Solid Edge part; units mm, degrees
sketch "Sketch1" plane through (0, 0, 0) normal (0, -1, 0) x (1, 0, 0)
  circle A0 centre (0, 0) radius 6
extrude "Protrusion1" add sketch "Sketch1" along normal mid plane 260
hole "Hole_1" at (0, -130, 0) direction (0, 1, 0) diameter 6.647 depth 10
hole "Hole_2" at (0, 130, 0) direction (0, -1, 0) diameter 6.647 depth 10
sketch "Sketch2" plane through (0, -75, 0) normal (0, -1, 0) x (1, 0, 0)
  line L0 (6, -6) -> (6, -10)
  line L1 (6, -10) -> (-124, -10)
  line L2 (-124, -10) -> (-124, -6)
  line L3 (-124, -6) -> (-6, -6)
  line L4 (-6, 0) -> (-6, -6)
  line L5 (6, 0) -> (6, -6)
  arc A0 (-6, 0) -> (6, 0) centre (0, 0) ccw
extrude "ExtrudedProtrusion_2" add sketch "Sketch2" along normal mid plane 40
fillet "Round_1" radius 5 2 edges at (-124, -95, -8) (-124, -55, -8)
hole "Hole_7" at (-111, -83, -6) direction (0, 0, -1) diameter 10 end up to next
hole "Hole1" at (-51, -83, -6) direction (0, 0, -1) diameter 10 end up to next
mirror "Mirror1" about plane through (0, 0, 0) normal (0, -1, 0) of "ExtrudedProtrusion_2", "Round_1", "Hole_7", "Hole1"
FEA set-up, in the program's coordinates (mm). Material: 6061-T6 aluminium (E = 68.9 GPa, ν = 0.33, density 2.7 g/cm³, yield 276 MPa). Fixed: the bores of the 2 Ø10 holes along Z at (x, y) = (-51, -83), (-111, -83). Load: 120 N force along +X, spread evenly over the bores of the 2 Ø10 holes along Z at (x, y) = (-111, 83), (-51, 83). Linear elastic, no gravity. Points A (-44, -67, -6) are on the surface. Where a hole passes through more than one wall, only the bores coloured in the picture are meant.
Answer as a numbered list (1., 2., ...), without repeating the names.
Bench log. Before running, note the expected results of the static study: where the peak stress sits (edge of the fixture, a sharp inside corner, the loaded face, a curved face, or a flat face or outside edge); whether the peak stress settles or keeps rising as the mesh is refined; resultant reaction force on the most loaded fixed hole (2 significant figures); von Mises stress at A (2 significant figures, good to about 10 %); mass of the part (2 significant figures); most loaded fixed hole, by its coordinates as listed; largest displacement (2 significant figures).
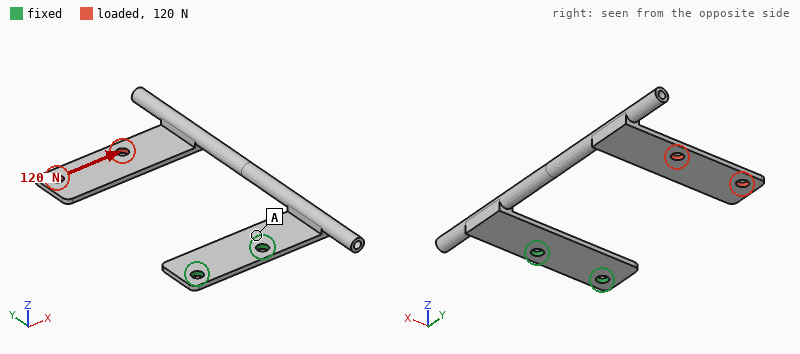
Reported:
1. a sharp inside corner
2. keeps rising
3. 360 N
4. 8.9 MPa
5. 190 g
6. (-111, -83)
7. 3.2 mm
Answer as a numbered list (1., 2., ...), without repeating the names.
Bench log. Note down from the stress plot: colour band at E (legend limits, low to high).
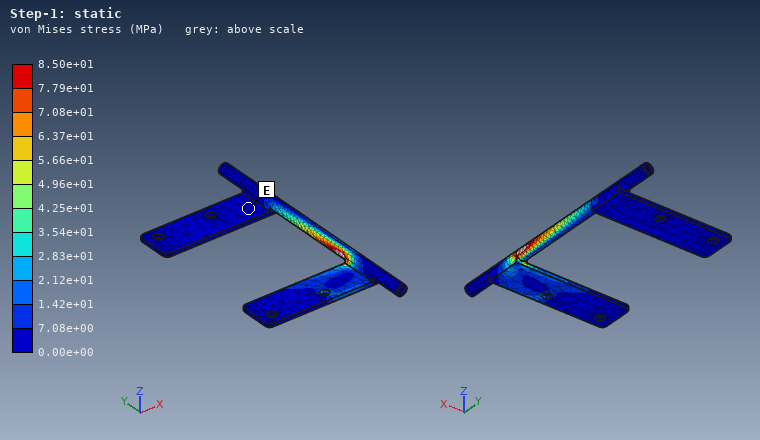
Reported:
1. 0.00e+00 to 7.08e+00 MPa
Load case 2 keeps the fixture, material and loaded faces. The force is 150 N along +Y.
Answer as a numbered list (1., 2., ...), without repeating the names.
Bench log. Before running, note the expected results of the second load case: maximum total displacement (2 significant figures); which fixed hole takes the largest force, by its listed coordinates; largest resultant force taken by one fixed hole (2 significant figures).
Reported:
1. 3.5 mm
2. (-51, -83)
3. 120 N
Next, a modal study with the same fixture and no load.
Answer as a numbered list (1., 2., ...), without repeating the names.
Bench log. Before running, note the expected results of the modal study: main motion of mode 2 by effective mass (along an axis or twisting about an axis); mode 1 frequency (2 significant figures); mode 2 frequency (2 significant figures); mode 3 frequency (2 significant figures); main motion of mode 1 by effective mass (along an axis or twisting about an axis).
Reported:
1. along X
2. 69 Hz
3. 120 Hz
4. 150 Hz
5. along Z
